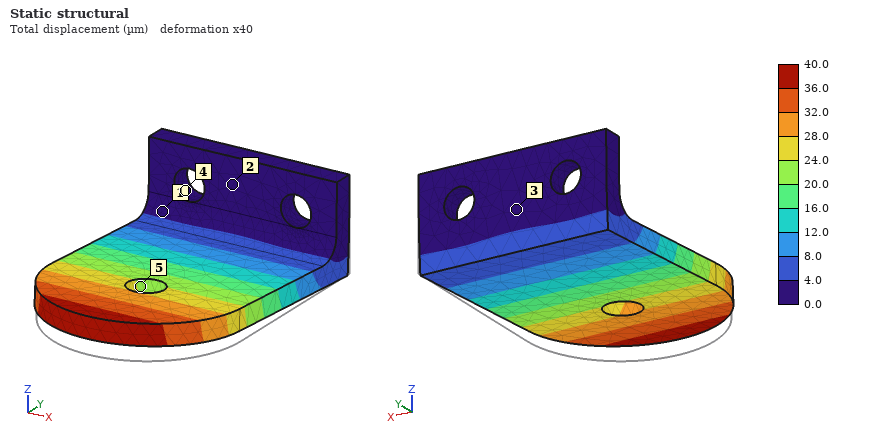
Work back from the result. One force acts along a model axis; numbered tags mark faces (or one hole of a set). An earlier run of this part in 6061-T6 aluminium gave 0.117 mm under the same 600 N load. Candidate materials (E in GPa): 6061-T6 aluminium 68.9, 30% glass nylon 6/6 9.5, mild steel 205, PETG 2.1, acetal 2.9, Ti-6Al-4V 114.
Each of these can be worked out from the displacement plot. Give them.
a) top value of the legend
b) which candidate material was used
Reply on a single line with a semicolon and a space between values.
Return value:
40.0 µm; mild steel
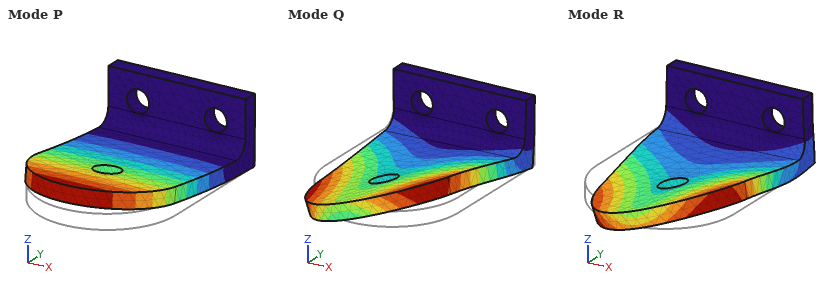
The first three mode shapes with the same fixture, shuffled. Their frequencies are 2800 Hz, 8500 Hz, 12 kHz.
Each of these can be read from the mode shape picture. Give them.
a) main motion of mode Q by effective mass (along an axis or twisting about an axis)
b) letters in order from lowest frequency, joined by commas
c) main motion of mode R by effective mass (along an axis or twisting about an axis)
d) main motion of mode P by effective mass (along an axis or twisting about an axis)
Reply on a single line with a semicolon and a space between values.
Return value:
along X; P, Q, R; along X; along Z
